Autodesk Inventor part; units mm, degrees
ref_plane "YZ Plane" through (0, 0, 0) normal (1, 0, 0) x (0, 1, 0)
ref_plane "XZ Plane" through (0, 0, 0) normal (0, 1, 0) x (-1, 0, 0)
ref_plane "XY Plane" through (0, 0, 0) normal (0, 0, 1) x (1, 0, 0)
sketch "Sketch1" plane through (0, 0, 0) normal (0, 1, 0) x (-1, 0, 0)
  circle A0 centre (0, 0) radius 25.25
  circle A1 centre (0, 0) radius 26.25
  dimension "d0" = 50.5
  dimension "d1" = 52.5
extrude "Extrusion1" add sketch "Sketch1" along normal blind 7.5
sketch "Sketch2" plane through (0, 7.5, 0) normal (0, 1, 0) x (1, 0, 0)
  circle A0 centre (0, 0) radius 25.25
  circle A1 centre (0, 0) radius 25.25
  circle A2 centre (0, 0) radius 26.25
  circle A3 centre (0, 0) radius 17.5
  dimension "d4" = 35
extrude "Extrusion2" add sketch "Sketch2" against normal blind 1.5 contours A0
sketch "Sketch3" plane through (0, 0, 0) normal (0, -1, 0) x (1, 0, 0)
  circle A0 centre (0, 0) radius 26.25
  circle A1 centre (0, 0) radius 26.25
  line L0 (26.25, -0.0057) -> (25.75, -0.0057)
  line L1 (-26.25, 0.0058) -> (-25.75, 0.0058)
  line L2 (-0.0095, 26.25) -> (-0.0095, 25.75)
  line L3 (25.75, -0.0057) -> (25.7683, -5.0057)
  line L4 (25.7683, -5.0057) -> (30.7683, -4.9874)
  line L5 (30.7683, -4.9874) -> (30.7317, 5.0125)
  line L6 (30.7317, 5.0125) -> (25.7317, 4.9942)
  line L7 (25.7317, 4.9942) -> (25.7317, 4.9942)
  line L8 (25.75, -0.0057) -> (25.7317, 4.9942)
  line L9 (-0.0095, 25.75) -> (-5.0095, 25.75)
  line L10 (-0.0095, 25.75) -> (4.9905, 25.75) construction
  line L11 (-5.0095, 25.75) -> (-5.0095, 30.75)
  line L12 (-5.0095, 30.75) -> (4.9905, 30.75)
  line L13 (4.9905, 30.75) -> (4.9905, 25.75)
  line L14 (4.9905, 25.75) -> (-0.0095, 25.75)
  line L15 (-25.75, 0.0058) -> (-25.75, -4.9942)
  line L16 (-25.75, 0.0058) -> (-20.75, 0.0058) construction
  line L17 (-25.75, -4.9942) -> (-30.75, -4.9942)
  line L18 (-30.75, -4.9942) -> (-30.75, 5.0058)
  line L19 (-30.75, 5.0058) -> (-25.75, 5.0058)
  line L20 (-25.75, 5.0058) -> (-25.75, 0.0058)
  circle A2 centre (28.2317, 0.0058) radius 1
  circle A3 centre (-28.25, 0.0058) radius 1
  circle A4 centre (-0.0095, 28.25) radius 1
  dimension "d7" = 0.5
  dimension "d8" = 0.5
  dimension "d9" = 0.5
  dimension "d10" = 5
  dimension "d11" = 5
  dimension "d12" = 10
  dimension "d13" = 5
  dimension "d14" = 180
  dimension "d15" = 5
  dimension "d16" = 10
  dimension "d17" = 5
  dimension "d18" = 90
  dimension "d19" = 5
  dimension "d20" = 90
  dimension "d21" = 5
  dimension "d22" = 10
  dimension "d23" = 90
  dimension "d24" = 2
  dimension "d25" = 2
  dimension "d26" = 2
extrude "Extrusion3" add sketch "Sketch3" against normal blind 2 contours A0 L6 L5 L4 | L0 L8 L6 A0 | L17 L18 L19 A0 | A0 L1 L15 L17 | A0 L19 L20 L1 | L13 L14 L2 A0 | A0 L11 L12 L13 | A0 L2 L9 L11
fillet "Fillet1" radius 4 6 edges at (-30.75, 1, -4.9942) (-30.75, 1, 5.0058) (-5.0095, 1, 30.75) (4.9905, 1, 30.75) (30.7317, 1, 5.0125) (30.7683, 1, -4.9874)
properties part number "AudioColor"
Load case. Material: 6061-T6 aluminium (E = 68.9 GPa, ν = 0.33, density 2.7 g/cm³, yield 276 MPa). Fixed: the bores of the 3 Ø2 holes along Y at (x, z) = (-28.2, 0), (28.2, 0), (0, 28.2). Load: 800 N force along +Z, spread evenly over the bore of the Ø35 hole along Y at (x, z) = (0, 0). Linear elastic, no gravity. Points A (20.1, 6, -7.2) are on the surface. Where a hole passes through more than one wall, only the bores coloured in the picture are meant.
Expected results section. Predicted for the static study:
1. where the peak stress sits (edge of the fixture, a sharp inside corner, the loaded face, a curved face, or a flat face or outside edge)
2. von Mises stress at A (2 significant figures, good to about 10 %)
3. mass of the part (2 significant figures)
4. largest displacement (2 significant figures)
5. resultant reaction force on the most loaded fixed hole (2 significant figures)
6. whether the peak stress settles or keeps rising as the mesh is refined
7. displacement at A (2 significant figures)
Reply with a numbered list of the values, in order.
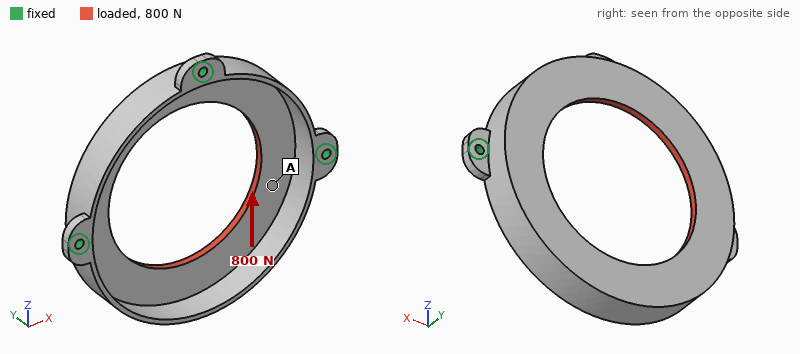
1. edge of the fixture
2. 18 MPa
3. 8.1 g
4. 0.11 mm
5. 320 N
6. keeps rising
7. 0.037 mm
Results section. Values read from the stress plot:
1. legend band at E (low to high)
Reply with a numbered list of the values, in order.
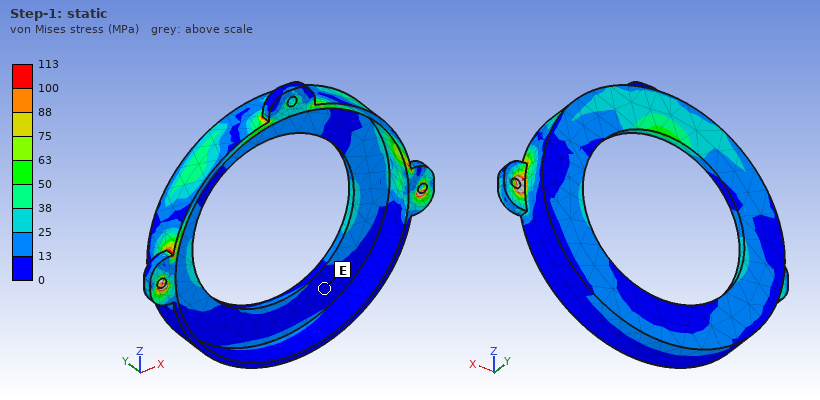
1. 0 to 13 MPa
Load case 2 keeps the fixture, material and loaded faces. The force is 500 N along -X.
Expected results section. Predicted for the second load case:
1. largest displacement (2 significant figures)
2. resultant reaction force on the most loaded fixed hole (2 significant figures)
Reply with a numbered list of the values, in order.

1. 0.10 mm
2. 190 N
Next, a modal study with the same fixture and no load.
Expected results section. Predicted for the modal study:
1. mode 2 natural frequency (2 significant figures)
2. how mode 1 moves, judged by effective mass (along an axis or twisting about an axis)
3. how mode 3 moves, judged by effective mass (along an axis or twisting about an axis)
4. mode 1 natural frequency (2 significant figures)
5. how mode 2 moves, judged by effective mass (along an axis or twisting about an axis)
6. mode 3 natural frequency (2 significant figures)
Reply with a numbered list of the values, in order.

1. 4700 Hz
2. along Y
3. along Z
4. 3100 Hz
5. along X
6. 9800 Hz
